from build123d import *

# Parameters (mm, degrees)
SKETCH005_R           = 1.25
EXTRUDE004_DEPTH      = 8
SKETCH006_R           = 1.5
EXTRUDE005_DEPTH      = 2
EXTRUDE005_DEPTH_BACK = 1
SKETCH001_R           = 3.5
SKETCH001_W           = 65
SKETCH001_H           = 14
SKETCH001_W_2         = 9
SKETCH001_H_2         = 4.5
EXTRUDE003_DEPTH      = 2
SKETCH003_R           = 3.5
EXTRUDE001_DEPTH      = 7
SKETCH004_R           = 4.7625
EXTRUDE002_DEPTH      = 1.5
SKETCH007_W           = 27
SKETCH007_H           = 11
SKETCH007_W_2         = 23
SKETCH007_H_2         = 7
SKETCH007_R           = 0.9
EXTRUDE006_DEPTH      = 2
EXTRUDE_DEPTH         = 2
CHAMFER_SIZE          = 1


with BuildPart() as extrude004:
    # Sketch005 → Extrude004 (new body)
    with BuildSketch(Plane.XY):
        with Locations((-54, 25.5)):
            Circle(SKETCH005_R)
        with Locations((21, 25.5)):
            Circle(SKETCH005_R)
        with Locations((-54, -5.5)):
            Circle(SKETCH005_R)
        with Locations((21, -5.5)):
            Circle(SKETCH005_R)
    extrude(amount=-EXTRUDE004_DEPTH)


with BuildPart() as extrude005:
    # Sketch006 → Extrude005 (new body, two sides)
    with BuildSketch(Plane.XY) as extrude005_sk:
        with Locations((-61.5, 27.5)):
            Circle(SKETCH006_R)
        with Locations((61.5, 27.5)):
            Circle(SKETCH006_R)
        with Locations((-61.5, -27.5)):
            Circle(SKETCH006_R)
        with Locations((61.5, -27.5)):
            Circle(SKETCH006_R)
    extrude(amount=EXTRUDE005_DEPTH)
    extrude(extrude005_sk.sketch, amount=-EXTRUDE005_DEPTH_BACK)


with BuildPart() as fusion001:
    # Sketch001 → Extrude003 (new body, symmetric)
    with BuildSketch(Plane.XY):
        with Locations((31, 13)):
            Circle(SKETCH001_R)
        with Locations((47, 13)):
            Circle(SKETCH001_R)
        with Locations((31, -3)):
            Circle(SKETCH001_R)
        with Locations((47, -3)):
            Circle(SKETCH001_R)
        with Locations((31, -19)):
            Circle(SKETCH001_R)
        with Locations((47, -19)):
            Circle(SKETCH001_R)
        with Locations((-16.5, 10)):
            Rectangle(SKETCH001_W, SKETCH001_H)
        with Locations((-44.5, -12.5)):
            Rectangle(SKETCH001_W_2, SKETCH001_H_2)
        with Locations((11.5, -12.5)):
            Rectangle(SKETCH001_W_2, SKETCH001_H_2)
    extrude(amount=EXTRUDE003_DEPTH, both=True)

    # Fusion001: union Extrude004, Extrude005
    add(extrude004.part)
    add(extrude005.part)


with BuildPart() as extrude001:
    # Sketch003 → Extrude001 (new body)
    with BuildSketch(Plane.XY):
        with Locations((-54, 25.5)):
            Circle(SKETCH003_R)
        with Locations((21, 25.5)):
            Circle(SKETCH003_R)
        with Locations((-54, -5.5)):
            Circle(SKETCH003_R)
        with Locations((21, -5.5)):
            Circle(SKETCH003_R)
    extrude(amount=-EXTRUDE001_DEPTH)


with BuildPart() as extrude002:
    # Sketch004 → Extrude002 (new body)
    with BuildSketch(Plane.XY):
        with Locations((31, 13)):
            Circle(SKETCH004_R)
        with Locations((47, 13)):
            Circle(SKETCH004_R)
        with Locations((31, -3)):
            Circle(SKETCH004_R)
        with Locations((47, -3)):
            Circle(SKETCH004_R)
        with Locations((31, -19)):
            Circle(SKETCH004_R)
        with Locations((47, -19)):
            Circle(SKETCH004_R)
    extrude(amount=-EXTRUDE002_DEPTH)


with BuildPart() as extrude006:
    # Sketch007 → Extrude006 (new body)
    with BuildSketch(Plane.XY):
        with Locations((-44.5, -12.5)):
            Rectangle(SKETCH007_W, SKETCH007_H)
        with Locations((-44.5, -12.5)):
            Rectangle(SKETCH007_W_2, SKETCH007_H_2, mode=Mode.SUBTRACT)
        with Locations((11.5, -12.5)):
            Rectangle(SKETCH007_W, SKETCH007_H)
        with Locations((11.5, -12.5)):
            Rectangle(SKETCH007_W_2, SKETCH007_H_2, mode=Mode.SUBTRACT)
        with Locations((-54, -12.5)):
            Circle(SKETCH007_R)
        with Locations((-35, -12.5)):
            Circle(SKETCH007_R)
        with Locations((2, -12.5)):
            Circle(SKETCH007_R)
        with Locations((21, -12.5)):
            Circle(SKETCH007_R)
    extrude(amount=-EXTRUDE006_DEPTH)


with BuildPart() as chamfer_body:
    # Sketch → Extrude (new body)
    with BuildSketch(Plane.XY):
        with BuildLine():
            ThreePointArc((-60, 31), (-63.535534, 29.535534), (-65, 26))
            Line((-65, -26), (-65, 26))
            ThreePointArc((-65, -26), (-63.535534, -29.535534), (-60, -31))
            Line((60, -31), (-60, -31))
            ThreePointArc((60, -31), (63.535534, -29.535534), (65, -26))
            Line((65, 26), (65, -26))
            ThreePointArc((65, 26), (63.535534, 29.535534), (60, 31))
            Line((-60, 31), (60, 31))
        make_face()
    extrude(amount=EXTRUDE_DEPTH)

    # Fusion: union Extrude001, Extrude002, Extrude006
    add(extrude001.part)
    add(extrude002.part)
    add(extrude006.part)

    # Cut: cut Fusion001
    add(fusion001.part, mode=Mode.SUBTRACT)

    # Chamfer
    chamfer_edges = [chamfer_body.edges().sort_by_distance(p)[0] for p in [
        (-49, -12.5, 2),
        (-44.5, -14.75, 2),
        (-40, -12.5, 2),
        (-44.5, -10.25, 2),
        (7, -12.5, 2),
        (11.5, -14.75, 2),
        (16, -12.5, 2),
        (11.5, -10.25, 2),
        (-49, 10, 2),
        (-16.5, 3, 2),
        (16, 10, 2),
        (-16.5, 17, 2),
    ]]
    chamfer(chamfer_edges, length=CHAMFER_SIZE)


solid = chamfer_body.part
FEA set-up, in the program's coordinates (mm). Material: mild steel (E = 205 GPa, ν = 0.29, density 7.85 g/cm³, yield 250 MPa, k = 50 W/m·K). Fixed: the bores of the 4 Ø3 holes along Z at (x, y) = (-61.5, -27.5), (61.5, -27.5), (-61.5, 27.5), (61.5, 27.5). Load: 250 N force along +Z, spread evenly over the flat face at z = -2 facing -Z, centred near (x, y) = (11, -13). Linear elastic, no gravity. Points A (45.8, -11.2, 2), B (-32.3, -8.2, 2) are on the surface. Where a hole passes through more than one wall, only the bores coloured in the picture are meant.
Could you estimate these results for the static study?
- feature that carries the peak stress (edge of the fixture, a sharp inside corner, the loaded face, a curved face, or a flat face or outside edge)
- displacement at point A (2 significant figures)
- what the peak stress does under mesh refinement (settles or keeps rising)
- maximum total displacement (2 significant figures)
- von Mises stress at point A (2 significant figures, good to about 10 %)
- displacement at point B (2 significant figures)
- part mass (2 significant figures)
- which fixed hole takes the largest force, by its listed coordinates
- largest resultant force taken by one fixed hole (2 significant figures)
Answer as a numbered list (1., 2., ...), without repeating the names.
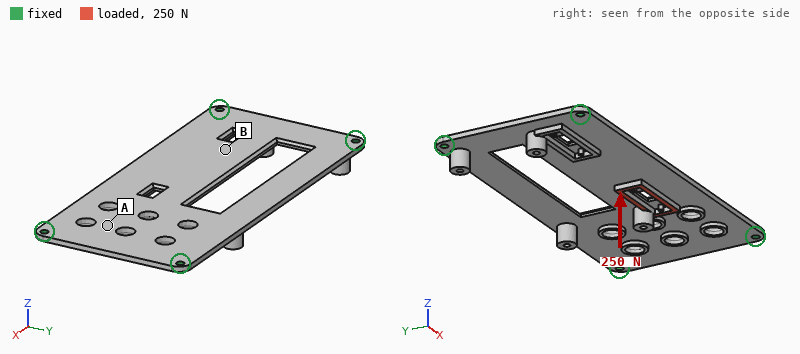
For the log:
1. edge of the fixture
2. 0.11 mm
3. keeps rising
4. 0.40 mm
5. 42 MPa
6. 0.21 mm
7. 120 g
8. (61.5, -27.5)
9. 130 N
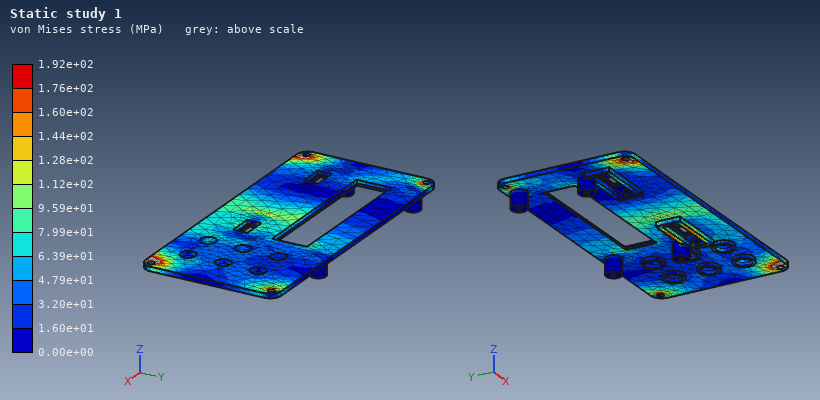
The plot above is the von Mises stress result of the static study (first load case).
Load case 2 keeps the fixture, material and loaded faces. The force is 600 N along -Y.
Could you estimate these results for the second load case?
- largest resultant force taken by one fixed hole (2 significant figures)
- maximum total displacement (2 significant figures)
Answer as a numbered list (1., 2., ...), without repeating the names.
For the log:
1. 360 N
2. 71 µm
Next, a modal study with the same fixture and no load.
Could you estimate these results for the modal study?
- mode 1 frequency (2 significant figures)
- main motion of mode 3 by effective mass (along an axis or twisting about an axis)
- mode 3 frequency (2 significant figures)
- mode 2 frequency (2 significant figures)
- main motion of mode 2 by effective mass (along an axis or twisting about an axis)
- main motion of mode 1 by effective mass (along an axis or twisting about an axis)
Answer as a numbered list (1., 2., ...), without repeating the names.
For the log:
1. 610 Hz
2. twisting about Y
3. 1700 Hz
4. 1000 Hz
5. twisting about X
6. along Z
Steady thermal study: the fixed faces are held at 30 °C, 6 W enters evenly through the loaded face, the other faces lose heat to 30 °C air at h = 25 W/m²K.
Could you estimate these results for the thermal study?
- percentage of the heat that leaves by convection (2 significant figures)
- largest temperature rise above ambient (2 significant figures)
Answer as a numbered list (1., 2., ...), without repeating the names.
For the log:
1. 66 %
2. 29 K
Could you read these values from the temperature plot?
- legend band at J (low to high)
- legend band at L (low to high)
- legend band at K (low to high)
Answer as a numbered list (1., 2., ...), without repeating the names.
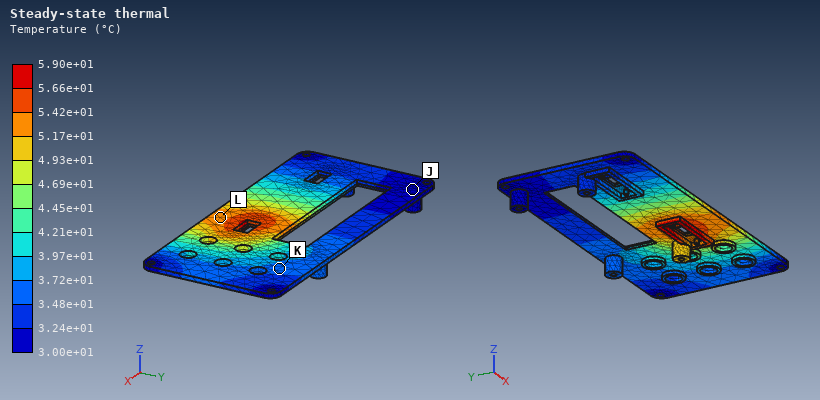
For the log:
1. 3.00e+01 to 3.24e+01 °C
2. 5.17e+01 to 5.42e+01 °C
3. 3.48e+01 to 3.72e+01 °C
